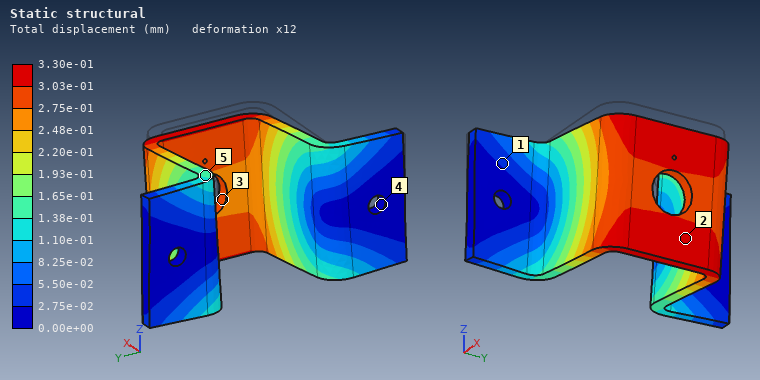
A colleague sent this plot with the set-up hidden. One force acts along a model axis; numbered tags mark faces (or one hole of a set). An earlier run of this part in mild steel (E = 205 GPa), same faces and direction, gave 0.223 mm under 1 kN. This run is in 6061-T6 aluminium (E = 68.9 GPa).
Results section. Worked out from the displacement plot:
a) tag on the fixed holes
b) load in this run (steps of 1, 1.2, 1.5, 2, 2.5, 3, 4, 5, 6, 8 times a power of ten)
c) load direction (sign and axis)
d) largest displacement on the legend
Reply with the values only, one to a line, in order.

4
500 N
-Z
3.30e-01 mm
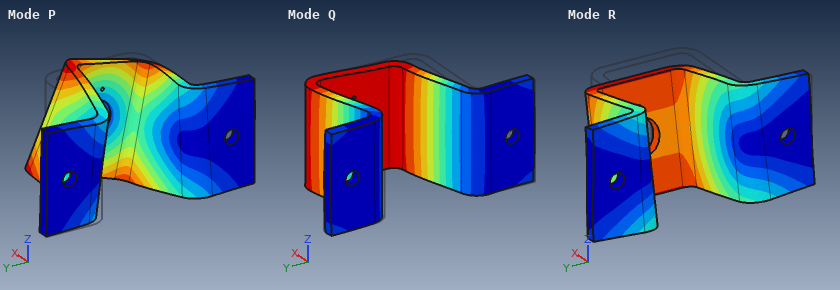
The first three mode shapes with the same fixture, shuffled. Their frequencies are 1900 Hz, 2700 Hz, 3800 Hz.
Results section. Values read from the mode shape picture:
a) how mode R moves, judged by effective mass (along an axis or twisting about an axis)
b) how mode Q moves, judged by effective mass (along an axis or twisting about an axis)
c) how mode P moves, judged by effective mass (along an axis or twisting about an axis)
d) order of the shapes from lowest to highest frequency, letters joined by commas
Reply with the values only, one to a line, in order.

along Z
along Y
twisting about X
R, Q, P
